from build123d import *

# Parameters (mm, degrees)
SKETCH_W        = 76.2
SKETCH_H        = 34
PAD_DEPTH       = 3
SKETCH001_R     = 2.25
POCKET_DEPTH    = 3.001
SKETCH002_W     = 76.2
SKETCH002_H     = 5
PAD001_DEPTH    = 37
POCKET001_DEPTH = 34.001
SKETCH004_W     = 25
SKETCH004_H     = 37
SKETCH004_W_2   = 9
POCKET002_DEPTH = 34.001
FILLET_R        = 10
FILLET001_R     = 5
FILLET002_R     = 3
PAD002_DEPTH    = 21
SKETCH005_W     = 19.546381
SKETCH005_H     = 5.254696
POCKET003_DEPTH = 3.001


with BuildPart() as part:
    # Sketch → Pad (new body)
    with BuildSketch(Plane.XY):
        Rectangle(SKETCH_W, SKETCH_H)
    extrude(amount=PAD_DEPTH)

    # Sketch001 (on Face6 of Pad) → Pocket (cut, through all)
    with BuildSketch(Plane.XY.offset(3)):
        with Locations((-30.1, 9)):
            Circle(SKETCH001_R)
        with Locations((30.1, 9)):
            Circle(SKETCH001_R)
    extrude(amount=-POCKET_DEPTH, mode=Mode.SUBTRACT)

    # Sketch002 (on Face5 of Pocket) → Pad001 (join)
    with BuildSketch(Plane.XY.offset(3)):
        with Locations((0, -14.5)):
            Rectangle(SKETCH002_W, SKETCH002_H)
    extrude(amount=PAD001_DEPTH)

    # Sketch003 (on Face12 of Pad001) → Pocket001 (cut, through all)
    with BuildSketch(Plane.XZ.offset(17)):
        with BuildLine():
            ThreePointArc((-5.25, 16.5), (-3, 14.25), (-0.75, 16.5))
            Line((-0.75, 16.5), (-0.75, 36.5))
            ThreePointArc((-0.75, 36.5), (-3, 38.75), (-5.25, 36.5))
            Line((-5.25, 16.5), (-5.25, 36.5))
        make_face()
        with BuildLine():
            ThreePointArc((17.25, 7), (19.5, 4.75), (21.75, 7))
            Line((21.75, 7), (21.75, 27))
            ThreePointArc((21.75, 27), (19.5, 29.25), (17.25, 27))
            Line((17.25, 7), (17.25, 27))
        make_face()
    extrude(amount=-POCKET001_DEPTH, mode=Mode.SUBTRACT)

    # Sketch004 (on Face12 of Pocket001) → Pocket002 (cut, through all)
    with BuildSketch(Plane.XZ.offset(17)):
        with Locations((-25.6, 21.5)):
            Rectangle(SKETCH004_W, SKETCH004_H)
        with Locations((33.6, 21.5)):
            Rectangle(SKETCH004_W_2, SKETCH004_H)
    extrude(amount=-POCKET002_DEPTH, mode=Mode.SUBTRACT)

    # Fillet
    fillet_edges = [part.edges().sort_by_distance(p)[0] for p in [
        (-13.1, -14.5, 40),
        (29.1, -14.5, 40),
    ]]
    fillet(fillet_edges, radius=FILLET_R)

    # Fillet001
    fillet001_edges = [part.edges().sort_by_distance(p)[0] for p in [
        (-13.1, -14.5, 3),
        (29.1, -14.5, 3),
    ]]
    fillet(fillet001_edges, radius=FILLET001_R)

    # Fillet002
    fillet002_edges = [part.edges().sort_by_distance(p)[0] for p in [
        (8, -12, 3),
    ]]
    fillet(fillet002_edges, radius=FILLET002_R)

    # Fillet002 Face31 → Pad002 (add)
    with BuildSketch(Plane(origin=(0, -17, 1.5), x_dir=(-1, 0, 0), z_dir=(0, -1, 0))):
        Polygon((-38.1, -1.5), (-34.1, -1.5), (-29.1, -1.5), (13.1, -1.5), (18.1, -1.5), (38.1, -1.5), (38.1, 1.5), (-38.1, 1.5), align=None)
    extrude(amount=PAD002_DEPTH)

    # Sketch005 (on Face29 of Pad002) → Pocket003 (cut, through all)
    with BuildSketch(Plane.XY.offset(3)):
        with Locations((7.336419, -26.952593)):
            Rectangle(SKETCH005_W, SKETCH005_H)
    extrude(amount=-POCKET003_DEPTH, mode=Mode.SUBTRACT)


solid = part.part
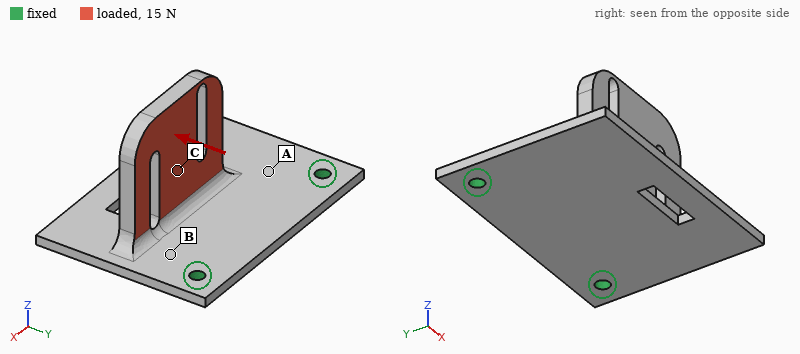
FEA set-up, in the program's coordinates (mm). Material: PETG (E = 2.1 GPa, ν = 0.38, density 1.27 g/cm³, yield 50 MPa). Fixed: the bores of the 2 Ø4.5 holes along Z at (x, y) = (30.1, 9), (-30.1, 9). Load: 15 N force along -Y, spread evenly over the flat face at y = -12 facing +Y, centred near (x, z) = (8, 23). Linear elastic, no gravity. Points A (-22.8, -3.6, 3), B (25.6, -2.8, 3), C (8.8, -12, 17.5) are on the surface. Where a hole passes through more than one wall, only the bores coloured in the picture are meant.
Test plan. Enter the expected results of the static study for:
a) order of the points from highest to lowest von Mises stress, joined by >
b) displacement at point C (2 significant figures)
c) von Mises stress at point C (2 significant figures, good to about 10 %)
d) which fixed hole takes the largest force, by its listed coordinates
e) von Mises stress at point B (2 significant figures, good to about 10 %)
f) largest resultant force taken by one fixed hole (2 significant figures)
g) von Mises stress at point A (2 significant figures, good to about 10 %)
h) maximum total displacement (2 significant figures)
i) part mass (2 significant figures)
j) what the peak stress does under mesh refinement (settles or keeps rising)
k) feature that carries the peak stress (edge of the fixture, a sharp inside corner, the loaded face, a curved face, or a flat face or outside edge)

B > A > C
0.46 mm
0.78 MPa
(30.1, 9)
3.2 MPa
9.9 N
2.3 MPa
1.1 mm
24 g
keeps rising
edge of the fixture
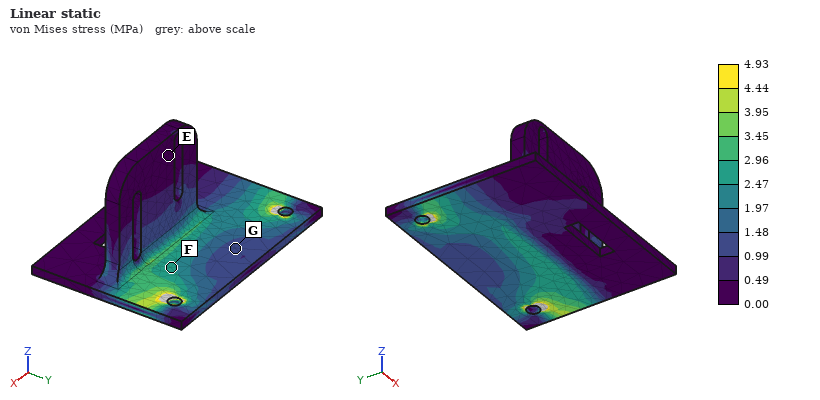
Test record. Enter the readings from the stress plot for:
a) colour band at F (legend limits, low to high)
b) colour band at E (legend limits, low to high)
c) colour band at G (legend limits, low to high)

2.47 to 2.96 MPa
0.00 to 0.49 MPa
0.99 to 1.48 MPa
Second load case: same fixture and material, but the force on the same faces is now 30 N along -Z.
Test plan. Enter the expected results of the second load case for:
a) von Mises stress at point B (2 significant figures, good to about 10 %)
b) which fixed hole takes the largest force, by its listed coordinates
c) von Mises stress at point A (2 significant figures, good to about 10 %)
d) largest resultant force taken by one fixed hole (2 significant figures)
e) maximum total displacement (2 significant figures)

3.0 MPa
(30.1, 9)
2.1 MPa
19 N
1.1 mm
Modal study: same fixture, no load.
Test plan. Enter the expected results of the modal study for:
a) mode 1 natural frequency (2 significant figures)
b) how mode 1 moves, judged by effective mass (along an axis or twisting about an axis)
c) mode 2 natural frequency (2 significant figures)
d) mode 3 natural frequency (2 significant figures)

180 Hz
along Z
450 Hz
640 Hz
